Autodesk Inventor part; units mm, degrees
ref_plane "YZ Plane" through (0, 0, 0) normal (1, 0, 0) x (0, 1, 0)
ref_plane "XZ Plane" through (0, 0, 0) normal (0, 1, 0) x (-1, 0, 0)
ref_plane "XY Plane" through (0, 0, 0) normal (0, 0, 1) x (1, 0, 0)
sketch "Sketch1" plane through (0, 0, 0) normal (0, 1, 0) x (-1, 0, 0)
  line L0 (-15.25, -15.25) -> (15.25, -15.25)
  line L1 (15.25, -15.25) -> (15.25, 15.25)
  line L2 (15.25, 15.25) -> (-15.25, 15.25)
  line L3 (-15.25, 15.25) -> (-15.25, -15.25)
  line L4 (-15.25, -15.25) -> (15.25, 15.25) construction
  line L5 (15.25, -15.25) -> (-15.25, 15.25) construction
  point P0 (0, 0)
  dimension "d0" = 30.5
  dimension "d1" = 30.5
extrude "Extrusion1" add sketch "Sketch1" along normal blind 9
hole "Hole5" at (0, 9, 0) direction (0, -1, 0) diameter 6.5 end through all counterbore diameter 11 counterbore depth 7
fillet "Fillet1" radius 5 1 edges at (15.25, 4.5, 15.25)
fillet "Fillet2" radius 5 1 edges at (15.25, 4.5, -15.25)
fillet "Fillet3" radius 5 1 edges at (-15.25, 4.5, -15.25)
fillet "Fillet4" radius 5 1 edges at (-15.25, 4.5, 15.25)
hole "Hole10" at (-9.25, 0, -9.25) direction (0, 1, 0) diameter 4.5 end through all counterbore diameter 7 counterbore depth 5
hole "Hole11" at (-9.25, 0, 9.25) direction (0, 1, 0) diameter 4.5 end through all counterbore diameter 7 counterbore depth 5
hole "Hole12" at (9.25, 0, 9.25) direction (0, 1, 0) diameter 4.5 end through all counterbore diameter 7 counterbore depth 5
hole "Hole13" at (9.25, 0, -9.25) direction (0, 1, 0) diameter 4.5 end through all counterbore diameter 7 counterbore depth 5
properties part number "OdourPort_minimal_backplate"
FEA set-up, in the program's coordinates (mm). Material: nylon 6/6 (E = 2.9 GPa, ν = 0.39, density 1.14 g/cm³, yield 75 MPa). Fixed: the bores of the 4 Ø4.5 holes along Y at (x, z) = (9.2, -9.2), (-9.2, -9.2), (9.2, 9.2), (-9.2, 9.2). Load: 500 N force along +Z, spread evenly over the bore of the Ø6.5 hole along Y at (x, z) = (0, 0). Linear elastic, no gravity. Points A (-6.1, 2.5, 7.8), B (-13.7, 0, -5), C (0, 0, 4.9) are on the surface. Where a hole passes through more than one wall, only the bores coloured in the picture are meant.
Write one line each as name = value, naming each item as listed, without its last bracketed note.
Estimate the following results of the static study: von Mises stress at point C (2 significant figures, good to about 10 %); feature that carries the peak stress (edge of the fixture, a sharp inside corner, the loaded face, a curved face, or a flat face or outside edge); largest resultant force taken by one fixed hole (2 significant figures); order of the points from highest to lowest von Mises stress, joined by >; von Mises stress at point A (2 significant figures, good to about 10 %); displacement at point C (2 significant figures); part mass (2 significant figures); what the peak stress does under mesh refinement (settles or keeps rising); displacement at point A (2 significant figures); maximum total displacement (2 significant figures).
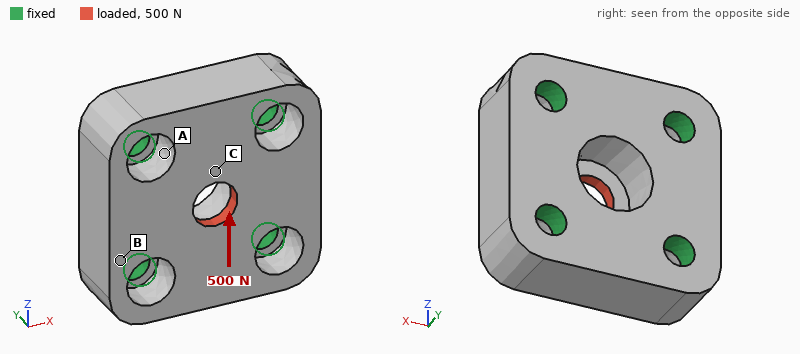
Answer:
von Mises stress at point C = 11 MPa
feature that carries the peak stress = a sharp inside corner
largest resultant force taken by one fixed hole = 140 N
order of the points from highest to lowest von Mises stress, joined by > = C > A > B
von Mises stress at point A = 4.4 MPa
displacement at point C = 36 µm
part mass = 7.3 g
what the peak stress does under mesh refinement = keeps rising
displacement at point A = 14 µm
maximum total displacement = 45 µm
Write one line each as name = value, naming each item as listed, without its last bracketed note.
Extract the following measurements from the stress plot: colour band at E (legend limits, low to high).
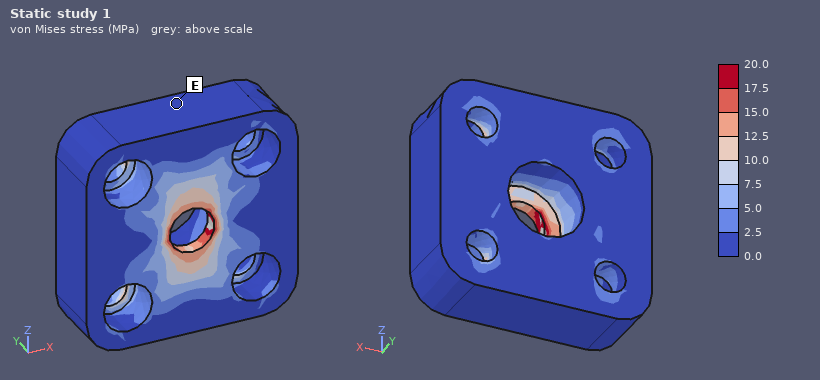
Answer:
colour band at E = 0.0 to 2.5 MPa
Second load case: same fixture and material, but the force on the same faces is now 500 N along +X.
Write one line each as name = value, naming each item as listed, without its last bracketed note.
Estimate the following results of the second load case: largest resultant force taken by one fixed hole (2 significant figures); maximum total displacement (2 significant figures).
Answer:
largest resultant force taken by one fixed hole = 140 N
maximum total displacement = 45 µm
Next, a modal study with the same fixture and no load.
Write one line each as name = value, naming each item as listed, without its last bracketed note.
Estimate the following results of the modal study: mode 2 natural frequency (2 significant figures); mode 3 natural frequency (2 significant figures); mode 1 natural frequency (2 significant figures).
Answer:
mode 2 natural frequency = 16 kHz
mode 3 natural frequency = 16 kHz
mode 1 natural frequency = 15 kHz
